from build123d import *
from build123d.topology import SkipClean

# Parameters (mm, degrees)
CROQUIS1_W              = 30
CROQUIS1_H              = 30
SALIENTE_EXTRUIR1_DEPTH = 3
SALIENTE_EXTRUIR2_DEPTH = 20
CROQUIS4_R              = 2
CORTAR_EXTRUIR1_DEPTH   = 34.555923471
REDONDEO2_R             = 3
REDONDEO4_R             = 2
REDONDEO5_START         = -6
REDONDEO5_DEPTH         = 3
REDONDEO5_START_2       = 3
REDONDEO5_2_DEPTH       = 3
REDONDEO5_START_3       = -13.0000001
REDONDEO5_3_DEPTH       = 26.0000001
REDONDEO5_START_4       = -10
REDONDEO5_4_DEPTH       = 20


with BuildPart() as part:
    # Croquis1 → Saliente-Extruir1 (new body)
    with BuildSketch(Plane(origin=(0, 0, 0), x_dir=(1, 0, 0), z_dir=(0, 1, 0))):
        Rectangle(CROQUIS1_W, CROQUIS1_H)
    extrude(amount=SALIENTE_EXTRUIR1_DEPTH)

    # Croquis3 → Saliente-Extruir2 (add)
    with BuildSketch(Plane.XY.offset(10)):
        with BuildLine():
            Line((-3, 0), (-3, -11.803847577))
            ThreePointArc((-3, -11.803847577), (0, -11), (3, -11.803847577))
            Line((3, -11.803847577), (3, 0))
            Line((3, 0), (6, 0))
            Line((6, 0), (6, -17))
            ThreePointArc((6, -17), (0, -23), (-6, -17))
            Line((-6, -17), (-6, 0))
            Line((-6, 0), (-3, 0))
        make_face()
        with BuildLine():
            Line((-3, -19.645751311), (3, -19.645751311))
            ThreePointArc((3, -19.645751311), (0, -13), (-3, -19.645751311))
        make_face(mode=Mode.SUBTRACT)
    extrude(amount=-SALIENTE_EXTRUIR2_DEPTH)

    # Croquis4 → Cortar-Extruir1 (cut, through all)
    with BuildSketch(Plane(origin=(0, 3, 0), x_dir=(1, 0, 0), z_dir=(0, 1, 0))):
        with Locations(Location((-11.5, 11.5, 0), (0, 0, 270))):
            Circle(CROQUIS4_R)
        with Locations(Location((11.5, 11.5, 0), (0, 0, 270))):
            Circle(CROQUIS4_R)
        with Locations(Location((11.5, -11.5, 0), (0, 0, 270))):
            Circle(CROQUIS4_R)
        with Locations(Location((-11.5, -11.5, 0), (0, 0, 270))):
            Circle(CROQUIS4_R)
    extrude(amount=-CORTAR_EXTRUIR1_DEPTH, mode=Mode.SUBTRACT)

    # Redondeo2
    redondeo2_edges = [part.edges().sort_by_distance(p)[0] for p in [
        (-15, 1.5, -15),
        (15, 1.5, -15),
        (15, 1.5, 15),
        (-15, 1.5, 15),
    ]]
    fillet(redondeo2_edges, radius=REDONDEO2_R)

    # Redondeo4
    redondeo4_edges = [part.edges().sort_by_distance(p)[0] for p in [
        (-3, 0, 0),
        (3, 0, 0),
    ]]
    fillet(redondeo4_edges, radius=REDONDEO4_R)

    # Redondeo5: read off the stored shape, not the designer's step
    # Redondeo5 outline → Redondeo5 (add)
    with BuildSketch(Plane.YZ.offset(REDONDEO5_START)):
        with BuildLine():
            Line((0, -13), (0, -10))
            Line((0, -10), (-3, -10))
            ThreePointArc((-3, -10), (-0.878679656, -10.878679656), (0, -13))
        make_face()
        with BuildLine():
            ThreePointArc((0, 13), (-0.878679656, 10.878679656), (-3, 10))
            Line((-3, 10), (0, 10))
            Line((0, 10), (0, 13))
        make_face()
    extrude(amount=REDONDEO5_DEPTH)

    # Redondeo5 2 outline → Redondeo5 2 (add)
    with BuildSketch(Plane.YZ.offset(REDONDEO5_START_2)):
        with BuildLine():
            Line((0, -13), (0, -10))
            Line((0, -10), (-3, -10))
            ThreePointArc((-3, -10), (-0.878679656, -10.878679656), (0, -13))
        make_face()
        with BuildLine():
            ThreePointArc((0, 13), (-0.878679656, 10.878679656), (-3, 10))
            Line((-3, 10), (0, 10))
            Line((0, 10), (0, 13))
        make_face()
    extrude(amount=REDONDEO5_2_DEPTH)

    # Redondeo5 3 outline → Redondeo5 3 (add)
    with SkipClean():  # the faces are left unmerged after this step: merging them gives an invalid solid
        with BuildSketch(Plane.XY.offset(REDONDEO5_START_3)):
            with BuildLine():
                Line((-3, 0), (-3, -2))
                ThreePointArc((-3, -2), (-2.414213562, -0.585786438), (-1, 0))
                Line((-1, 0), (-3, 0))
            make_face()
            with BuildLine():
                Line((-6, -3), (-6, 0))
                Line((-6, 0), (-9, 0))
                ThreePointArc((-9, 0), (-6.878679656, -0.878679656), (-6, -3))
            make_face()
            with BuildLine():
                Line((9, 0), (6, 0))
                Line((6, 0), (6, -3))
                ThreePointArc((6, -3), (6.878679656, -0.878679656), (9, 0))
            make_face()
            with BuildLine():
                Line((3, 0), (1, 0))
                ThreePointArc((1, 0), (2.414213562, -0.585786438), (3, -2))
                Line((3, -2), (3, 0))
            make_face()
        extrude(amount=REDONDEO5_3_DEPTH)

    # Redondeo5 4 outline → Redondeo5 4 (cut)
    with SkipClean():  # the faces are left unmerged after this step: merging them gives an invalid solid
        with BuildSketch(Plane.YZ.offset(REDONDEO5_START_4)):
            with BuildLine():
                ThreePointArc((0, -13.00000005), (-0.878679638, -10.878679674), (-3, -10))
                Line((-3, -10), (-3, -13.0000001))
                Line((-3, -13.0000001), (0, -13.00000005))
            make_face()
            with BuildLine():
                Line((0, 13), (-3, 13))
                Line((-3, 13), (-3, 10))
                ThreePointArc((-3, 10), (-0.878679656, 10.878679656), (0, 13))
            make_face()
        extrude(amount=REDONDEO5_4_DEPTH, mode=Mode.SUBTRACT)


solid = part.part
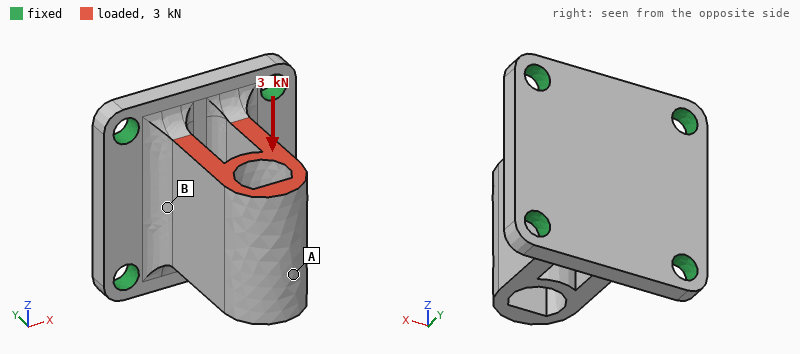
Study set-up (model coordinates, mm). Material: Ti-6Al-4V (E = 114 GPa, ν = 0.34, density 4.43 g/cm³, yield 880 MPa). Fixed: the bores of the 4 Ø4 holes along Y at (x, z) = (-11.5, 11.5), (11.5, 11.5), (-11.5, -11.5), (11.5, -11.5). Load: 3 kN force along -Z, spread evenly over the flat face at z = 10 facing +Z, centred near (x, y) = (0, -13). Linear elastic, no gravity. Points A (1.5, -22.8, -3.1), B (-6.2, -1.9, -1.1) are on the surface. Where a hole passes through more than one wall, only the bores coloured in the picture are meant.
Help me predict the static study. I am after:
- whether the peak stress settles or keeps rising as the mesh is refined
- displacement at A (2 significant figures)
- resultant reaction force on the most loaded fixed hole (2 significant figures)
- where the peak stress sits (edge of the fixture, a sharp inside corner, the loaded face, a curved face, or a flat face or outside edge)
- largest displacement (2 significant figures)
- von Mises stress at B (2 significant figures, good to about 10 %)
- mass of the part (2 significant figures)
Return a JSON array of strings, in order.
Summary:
["keeps rising", "50 µm", "1.3 kN", "edge of the fixture", "56 µm", "58 MPa", "25 g"]
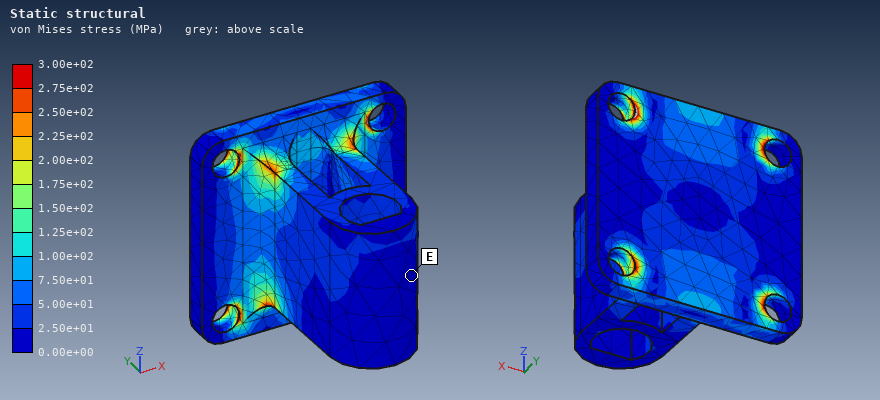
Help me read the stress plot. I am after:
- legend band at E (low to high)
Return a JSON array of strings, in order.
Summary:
["0.00e+00 to 2.50e+01 MPa"]
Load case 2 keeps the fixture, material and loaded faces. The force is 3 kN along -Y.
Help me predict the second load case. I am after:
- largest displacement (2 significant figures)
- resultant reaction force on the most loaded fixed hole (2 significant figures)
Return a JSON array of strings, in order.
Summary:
["57 µm", "1.5 kN"]
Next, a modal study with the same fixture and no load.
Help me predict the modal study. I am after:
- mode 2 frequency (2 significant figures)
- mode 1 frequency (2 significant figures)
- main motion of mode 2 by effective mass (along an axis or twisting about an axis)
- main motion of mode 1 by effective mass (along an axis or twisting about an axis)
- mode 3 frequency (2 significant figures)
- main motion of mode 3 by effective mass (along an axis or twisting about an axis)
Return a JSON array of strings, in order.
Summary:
["13 kHz", "8600 Hz", "along Z", "along X", "17 kHz", "along Y"]
